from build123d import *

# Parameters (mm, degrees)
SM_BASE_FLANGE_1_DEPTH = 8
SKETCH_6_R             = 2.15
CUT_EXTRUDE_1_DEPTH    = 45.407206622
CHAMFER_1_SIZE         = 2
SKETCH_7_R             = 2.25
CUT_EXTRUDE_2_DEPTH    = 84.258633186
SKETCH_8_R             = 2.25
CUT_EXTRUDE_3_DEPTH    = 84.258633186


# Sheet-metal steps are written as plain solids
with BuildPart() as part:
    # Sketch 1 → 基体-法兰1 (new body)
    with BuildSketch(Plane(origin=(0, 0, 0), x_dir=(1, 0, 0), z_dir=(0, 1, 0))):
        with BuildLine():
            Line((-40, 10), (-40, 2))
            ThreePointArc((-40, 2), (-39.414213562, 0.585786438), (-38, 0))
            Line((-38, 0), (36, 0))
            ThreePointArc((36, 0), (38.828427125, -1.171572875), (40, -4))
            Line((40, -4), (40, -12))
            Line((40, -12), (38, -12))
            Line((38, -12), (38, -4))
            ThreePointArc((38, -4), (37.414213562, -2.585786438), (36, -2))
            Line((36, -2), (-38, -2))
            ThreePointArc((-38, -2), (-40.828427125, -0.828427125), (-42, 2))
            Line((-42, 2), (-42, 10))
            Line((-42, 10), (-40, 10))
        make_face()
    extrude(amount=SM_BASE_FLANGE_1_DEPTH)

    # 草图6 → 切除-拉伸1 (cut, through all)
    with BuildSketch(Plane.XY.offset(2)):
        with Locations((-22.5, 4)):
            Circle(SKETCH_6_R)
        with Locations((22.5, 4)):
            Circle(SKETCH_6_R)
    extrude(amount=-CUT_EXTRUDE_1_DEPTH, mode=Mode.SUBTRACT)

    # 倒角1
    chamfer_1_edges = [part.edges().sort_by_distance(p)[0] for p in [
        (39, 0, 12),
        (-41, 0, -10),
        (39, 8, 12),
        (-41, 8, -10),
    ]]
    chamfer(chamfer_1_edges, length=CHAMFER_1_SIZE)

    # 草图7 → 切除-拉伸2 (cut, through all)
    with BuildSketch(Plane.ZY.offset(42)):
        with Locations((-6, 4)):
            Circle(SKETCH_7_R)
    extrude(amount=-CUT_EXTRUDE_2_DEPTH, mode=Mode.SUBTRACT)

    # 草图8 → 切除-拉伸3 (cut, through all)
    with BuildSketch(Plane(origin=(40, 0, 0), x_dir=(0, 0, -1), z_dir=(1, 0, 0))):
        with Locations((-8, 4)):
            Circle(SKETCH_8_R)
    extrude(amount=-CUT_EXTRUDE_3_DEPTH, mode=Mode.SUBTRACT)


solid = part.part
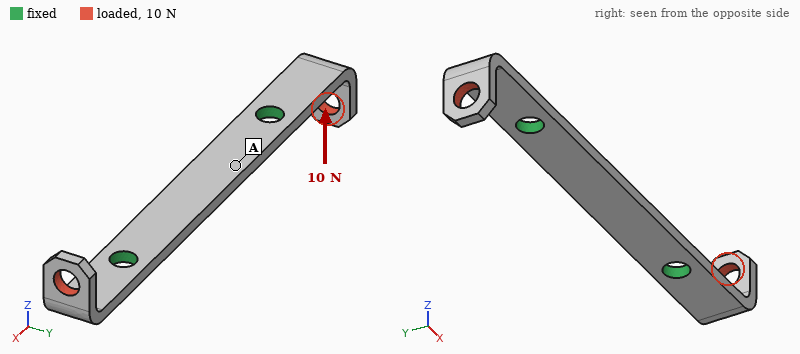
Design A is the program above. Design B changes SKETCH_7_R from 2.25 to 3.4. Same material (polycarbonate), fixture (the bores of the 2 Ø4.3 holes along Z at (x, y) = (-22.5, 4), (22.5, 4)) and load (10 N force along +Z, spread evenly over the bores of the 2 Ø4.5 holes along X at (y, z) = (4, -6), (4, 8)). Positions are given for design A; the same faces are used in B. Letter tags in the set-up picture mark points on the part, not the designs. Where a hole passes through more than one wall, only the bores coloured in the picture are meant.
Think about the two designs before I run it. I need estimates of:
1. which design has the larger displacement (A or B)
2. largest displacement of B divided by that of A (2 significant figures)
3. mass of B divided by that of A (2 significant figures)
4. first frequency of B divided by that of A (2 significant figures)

B
1.2
0.97
1.2
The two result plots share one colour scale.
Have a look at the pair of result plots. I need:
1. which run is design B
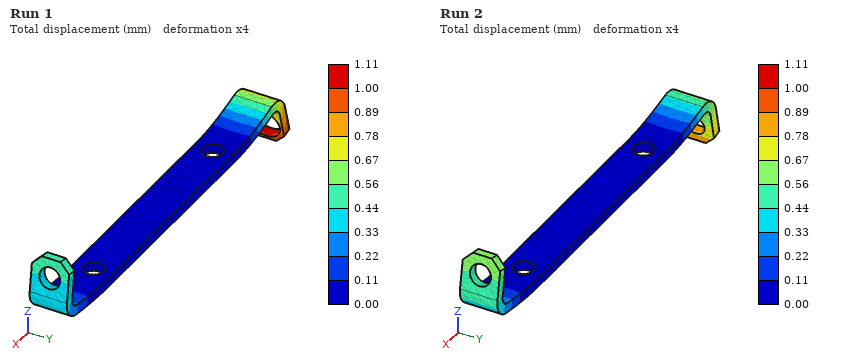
Run 1
